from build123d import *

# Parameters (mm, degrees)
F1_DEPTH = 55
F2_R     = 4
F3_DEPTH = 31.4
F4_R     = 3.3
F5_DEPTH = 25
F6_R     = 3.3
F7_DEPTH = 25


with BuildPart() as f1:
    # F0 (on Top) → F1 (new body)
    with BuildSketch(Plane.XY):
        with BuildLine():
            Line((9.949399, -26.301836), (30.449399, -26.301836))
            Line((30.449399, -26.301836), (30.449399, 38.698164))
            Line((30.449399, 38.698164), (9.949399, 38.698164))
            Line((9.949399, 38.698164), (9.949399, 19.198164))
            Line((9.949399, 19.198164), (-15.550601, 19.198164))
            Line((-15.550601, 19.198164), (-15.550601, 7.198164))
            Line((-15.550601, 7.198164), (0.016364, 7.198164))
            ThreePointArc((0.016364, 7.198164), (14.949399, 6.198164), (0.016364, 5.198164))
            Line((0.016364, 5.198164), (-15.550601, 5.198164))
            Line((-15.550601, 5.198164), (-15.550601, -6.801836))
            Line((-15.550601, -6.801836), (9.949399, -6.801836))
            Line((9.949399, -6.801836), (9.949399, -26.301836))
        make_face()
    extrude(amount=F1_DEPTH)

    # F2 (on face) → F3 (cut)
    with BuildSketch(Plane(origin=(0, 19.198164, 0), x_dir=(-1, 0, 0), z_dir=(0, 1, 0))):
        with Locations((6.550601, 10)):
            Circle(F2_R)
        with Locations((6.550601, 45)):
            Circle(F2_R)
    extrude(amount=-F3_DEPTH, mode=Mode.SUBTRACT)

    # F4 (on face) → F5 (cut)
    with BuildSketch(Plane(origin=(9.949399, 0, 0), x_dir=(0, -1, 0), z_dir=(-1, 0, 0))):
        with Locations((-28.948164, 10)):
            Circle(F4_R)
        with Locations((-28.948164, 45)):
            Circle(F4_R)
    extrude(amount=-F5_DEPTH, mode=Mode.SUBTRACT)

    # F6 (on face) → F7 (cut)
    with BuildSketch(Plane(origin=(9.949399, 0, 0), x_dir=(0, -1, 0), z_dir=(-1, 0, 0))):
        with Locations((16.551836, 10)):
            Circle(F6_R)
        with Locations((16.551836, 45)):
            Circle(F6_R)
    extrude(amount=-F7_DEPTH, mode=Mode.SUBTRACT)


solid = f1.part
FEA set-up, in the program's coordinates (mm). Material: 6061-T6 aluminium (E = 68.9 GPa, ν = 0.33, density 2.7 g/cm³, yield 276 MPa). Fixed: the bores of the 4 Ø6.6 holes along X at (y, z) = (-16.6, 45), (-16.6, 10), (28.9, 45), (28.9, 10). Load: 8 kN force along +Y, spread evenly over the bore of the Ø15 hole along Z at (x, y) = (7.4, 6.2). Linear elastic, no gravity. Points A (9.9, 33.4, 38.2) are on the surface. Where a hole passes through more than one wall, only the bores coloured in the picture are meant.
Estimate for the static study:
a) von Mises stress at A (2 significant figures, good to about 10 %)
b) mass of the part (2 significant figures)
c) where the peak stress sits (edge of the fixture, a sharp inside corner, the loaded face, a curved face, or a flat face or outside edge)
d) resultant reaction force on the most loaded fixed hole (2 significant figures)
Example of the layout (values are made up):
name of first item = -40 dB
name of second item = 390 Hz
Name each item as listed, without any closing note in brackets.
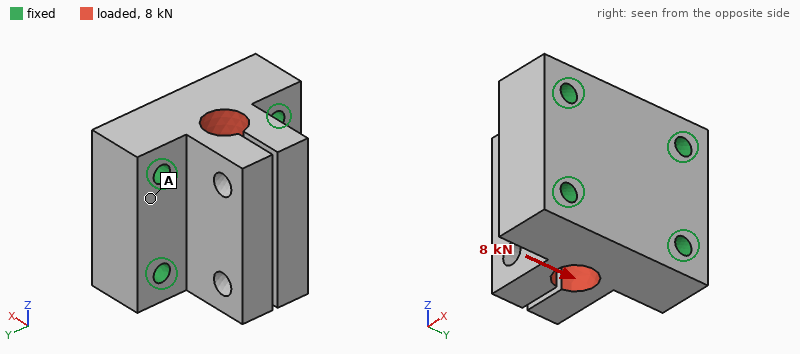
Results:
von Mises stress at A = 4.2 MPa
mass of the part = 250 g
where the peak stress sits = the loaded face
resultant reaction force on the most loaded fixed hole = 2.2 kN
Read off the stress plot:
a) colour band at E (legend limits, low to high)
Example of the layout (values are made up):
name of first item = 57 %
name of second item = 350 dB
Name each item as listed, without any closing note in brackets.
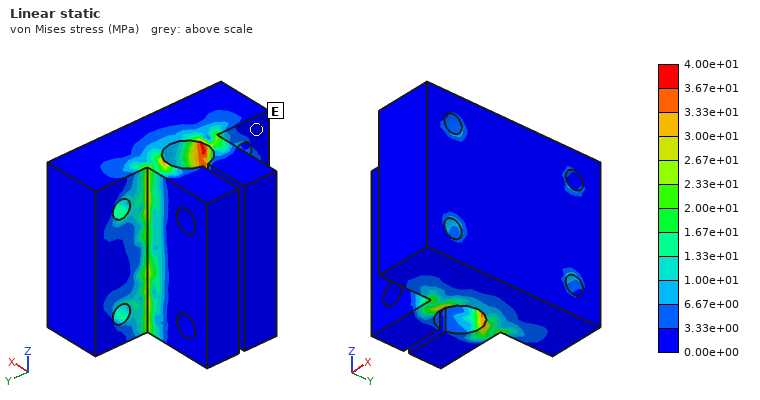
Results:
colour band at E = 0.00e+00 to 3.33e+00 MPa
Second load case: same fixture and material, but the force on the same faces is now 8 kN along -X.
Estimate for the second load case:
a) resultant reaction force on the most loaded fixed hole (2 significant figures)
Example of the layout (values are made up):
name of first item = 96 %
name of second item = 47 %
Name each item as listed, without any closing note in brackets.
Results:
resultant reaction force on the most loaded fixed hole = 2.0 kN
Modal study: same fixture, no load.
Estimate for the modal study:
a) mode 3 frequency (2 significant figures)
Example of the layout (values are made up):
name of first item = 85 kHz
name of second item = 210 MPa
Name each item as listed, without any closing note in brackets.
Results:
mode 3 frequency = 9300 Hz
